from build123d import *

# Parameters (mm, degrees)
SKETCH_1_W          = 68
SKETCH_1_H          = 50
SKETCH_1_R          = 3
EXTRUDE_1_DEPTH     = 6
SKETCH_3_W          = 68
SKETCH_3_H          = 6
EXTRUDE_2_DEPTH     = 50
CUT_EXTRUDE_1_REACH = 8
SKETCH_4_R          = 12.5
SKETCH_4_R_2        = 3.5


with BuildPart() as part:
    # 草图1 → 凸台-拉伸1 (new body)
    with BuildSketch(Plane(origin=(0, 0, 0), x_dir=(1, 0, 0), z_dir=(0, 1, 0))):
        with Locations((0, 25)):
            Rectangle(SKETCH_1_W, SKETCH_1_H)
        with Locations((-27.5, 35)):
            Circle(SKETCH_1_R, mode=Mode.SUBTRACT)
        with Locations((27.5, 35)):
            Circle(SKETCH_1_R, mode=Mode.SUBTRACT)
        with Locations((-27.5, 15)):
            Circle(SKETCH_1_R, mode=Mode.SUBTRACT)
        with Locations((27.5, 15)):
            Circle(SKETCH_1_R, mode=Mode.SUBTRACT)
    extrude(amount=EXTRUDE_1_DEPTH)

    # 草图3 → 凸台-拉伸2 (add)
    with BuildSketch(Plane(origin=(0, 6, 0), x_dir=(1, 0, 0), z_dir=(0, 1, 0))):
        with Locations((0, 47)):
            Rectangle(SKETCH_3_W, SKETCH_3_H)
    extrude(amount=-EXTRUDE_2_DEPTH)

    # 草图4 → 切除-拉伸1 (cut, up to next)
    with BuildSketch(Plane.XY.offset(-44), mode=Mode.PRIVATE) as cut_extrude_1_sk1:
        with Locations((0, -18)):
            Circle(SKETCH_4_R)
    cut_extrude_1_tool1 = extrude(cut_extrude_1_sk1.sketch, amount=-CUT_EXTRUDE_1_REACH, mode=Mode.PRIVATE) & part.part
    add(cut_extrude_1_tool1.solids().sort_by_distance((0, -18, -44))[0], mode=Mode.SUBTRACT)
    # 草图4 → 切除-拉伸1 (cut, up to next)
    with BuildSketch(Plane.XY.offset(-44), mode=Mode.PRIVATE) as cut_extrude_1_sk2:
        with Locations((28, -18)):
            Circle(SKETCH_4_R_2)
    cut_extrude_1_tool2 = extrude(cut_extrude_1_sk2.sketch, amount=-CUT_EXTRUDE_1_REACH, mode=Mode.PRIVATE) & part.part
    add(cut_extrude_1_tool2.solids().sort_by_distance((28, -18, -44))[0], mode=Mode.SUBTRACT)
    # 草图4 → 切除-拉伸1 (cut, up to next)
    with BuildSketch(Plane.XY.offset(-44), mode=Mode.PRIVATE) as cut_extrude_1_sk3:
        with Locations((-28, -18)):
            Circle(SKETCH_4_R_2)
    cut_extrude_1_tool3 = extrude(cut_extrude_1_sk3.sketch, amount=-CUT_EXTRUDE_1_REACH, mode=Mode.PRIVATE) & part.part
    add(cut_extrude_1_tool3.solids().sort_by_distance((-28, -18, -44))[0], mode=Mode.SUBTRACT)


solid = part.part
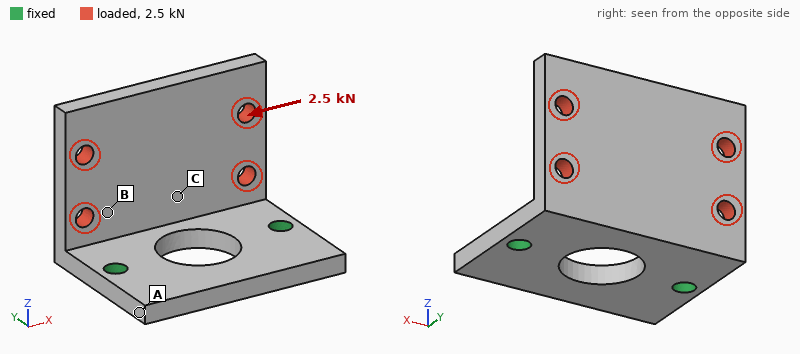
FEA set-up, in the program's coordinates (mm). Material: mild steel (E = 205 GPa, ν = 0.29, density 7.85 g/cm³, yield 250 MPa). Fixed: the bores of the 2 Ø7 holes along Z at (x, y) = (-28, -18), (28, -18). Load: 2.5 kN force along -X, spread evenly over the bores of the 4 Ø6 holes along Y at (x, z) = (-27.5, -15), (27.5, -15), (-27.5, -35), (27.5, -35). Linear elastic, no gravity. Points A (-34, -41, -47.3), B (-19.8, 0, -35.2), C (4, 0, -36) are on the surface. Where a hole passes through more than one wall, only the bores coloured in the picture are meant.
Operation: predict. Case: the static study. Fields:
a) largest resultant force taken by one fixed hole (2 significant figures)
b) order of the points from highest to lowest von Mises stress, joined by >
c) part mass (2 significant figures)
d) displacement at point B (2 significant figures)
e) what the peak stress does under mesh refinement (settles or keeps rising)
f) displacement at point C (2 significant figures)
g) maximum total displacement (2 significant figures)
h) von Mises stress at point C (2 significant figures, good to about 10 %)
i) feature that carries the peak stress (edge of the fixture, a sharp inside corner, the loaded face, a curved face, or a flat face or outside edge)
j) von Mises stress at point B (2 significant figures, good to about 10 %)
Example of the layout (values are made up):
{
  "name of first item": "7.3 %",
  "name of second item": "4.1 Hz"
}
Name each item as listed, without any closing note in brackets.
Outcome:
{
  "largest resultant force taken by one fixed hole": "1.8 kN",
  "order of the points from highest to lowest von Mises stress, joined by >": "B > C > A",
  "part mass": "270 g",
  "displacement at point B": "19 µm",
  "what the peak stress does under mesh refinement": "keeps rising",
  "displacement at point C": "12 µm",
  "maximum total displacement": "49 µm",
  "von Mises stress at point C": "25 MPa",
  "feature that carries the peak stress": "edge of the fixture",
  "von Mises stress at point B": "36 MPa"
}
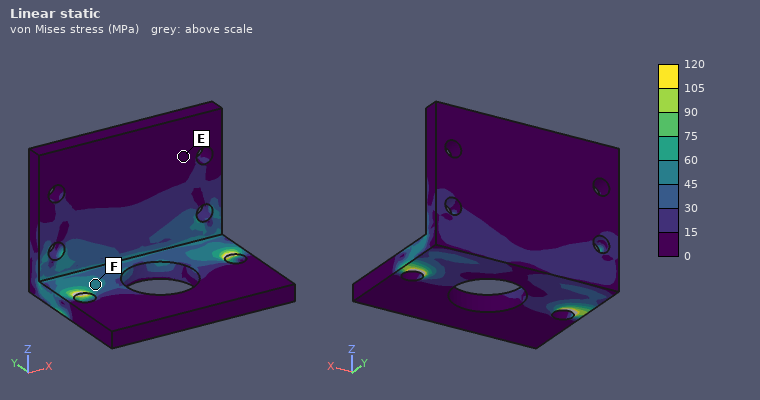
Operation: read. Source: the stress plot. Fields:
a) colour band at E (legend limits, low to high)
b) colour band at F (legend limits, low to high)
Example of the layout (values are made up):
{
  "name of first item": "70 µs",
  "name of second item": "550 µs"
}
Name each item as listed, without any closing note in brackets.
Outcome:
{
  "colour band at E": "0 to 15 MPa",
  "colour band at F": "45 to 60 MPa"
}
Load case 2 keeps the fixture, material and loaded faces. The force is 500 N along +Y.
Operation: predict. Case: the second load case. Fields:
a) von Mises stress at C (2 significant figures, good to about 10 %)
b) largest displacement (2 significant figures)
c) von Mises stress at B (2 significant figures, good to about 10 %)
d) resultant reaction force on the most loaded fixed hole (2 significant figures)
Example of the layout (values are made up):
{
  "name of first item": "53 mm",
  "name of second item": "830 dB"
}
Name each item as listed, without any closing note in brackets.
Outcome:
{
  "von Mises stress at C": "14 MPa",
  "largest displacement": "76 µm",
  "von Mises stress at B": "15 MPa",
  "resultant reaction force on the most loaded fixed hole": "250 N"
}
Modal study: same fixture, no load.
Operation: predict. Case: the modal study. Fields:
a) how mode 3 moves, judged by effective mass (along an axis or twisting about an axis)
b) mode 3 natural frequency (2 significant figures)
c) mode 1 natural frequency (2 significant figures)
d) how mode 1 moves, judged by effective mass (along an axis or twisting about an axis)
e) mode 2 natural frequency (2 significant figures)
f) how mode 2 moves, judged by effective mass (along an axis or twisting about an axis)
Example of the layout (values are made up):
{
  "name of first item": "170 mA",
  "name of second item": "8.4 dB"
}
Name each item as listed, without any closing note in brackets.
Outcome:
{
  "how mode 3 moves, judged by effective mass": "along Z",
  "mode 3 natural frequency": "4300 Hz",
  "mode 1 natural frequency": "1200 Hz",
  "how mode 1 moves, judged by effective mass": "along Y",
  "mode 2 natural frequency": "2900 Hz",
  "how mode 2 moves, judged by effective mass": "along X"
}
